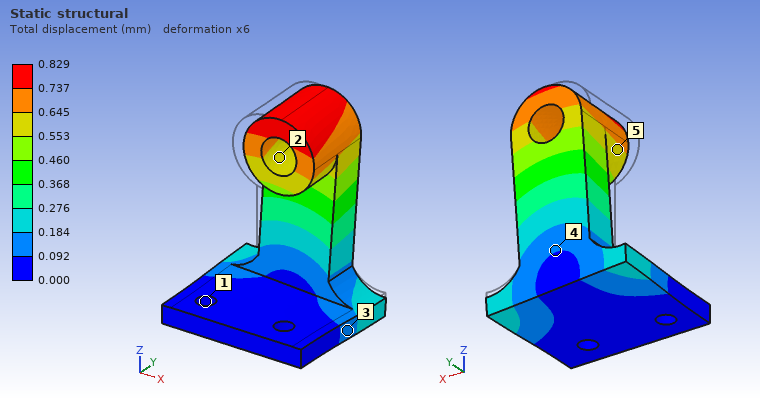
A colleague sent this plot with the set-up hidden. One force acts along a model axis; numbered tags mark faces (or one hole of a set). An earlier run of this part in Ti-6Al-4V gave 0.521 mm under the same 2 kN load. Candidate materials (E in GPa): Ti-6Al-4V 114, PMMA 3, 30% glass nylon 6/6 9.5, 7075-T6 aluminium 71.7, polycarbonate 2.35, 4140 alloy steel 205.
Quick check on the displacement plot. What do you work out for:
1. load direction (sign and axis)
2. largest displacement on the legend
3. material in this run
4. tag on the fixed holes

+X
0.829 mm
7075-T6 aluminium
1
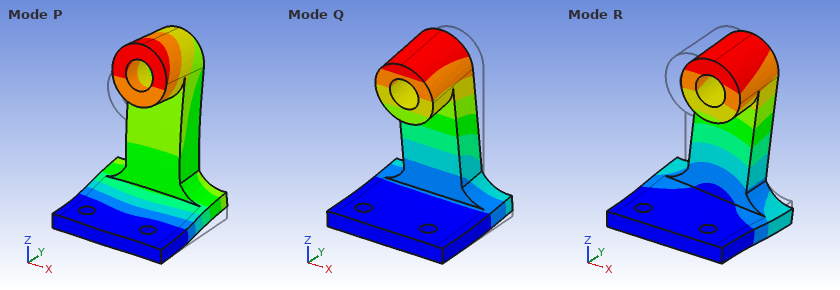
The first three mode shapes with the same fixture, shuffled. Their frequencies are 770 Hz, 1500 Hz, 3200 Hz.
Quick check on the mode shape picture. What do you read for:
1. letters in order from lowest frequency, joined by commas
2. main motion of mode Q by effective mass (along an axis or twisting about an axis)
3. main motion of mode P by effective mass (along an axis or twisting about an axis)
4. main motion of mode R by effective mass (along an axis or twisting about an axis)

Q, R, P
along Y
along Z
along X
